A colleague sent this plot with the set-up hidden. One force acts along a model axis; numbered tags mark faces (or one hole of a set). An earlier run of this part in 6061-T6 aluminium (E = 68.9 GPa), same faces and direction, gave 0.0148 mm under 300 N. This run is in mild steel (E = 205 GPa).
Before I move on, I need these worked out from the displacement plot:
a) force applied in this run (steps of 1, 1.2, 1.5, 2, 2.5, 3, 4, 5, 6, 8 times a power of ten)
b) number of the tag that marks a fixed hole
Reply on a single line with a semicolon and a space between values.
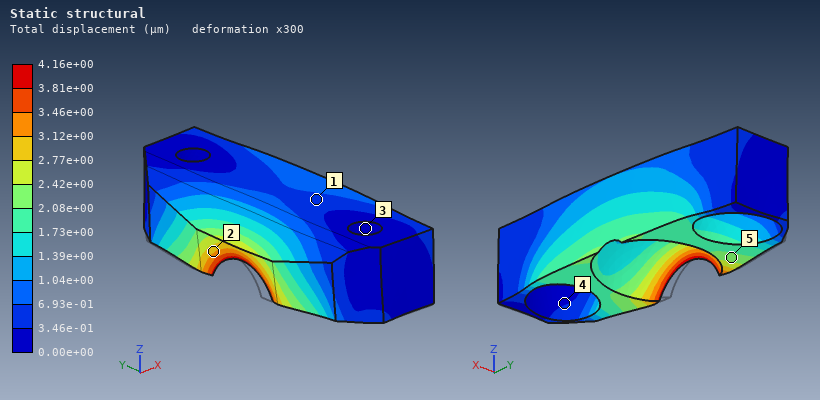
250 N; 3
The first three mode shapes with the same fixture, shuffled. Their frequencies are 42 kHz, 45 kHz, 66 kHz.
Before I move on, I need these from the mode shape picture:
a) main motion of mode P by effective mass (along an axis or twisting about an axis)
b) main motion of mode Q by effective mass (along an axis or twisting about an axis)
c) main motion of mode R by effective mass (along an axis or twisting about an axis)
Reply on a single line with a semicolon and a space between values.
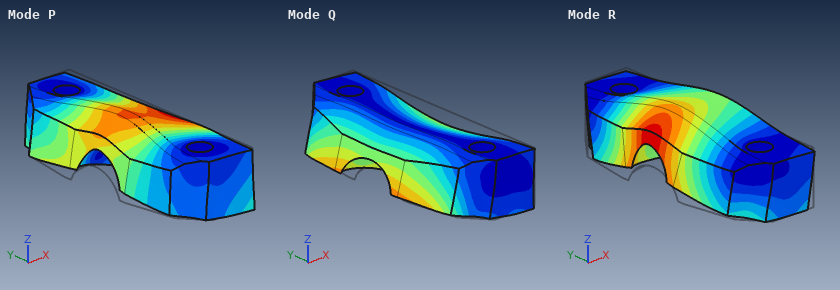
along X; along X; along Z
